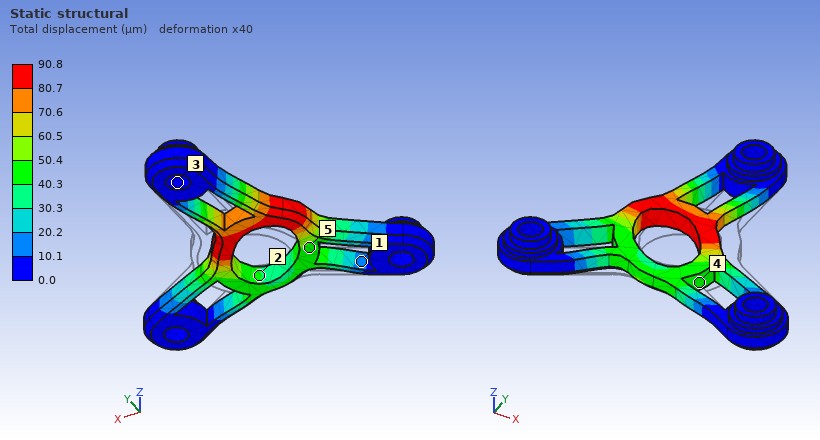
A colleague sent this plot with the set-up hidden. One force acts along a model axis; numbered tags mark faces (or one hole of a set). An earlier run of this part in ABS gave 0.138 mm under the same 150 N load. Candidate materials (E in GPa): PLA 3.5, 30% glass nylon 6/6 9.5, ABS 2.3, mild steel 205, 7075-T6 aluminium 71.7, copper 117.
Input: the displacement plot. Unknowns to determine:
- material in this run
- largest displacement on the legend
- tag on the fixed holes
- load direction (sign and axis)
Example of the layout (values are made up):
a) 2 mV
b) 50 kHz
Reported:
a) PLA
b) 90.8 µm
c) 3
d) -X
